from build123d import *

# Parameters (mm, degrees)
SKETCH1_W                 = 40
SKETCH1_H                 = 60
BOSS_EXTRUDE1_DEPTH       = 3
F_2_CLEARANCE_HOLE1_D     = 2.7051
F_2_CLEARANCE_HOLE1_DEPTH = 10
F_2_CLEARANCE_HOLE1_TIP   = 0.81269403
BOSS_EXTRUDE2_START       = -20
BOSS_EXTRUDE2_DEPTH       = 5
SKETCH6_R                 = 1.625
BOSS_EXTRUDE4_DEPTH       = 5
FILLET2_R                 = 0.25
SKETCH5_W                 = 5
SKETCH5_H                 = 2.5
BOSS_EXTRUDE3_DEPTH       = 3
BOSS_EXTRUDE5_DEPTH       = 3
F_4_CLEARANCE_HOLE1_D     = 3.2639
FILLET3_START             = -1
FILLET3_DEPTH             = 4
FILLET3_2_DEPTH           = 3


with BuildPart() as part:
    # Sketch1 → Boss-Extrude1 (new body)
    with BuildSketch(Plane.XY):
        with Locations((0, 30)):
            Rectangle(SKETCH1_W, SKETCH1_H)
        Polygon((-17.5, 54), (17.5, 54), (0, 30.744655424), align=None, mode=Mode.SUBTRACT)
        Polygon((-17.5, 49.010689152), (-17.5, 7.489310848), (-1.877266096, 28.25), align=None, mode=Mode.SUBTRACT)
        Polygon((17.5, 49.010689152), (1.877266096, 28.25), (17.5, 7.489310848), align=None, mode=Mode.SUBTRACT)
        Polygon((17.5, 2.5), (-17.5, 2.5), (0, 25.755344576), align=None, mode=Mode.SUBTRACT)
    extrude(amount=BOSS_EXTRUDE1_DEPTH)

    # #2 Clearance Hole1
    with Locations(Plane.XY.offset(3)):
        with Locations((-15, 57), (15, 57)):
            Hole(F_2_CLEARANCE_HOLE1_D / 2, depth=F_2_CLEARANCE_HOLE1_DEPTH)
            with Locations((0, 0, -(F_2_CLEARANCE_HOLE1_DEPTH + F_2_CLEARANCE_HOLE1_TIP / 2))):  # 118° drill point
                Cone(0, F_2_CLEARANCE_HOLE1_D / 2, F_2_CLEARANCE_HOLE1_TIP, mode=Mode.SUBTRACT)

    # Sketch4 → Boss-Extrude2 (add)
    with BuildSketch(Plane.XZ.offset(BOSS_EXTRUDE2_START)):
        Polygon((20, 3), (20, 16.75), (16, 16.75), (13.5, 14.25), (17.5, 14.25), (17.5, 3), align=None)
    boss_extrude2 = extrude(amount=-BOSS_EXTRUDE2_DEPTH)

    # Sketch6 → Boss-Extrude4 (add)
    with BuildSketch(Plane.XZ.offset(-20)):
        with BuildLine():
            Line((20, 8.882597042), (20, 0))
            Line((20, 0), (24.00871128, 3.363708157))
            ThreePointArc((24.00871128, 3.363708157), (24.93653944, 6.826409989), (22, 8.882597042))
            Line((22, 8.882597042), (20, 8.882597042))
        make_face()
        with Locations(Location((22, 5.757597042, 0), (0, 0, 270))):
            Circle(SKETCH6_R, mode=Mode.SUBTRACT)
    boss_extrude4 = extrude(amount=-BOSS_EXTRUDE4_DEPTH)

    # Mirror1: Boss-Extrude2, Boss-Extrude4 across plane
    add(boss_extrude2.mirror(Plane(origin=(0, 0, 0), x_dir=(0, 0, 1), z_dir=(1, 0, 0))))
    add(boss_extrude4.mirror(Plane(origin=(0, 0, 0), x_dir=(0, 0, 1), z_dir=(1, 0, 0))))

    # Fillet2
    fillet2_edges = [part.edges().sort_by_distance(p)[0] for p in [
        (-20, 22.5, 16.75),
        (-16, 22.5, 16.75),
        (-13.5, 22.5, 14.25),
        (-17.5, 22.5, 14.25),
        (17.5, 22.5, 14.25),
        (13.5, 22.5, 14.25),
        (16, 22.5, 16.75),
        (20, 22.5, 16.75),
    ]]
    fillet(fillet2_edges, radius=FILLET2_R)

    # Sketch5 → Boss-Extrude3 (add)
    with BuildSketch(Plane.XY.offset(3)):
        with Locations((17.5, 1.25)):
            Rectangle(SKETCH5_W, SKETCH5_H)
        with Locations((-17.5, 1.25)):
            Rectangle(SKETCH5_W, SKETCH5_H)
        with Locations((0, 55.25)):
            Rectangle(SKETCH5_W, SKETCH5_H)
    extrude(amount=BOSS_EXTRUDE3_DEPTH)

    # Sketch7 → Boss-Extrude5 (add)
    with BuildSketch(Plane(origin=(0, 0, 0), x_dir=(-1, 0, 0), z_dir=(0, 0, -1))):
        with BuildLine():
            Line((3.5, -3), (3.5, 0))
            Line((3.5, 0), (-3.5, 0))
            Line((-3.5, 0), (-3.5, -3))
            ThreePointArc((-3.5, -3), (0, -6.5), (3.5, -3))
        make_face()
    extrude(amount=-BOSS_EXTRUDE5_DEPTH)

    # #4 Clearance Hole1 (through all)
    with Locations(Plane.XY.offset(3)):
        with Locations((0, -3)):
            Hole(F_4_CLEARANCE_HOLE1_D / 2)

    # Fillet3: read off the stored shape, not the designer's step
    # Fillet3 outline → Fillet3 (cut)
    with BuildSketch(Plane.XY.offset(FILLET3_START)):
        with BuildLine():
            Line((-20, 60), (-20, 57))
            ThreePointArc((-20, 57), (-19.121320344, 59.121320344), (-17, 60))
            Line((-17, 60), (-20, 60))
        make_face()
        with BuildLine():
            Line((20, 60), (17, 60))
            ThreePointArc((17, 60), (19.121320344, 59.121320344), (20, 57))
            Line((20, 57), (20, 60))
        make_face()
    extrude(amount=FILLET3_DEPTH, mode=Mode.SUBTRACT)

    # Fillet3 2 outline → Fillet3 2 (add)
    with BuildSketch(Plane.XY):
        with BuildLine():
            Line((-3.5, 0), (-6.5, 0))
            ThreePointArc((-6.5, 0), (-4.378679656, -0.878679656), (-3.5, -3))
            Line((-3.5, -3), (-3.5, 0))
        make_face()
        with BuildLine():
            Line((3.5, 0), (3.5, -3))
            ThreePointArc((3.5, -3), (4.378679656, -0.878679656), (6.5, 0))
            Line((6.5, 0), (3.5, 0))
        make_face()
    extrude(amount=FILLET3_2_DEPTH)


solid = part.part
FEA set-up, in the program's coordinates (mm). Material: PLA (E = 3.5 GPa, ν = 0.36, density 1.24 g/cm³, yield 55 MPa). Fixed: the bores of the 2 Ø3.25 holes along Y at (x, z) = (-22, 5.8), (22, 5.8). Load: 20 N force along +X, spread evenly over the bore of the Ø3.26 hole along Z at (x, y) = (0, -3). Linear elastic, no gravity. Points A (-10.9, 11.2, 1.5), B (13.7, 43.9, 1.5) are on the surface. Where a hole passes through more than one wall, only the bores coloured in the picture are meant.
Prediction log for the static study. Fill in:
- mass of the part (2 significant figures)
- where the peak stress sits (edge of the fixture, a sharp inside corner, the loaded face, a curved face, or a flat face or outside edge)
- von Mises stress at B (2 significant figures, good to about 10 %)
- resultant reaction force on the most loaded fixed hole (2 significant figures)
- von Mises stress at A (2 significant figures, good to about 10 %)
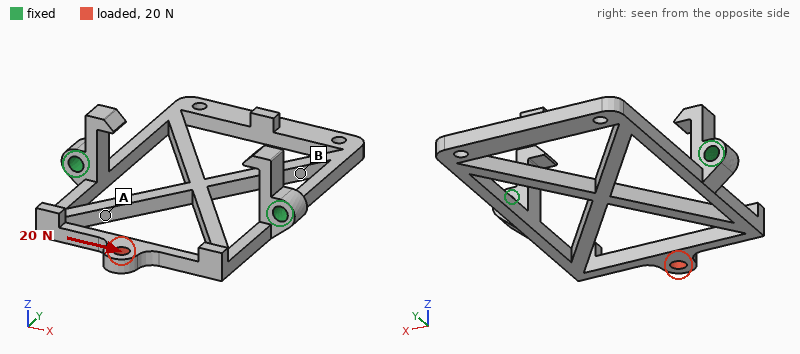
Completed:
4.5 g
a flat face or outside edge
1.7 MPa
15 N
6.0 MPa
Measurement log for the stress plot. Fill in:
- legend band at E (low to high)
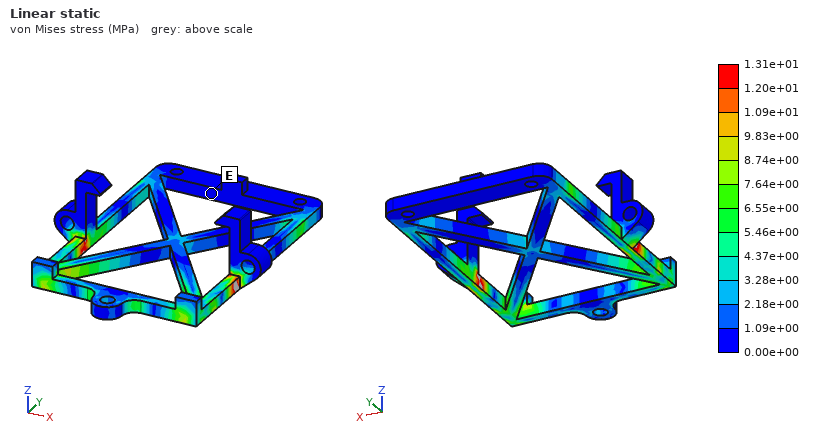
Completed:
0.00e+00 to 1.09e+00 MPa
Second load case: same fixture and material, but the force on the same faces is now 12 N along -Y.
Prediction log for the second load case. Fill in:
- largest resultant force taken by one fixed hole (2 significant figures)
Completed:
6.3 N
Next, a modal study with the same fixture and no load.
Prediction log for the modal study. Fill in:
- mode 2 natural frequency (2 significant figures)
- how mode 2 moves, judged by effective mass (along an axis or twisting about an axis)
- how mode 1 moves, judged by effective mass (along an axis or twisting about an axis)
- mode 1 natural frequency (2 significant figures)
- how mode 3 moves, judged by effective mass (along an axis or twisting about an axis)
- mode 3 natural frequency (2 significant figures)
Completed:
690 Hz
along Z
along Z
300 Hz
along X
740 Hz
